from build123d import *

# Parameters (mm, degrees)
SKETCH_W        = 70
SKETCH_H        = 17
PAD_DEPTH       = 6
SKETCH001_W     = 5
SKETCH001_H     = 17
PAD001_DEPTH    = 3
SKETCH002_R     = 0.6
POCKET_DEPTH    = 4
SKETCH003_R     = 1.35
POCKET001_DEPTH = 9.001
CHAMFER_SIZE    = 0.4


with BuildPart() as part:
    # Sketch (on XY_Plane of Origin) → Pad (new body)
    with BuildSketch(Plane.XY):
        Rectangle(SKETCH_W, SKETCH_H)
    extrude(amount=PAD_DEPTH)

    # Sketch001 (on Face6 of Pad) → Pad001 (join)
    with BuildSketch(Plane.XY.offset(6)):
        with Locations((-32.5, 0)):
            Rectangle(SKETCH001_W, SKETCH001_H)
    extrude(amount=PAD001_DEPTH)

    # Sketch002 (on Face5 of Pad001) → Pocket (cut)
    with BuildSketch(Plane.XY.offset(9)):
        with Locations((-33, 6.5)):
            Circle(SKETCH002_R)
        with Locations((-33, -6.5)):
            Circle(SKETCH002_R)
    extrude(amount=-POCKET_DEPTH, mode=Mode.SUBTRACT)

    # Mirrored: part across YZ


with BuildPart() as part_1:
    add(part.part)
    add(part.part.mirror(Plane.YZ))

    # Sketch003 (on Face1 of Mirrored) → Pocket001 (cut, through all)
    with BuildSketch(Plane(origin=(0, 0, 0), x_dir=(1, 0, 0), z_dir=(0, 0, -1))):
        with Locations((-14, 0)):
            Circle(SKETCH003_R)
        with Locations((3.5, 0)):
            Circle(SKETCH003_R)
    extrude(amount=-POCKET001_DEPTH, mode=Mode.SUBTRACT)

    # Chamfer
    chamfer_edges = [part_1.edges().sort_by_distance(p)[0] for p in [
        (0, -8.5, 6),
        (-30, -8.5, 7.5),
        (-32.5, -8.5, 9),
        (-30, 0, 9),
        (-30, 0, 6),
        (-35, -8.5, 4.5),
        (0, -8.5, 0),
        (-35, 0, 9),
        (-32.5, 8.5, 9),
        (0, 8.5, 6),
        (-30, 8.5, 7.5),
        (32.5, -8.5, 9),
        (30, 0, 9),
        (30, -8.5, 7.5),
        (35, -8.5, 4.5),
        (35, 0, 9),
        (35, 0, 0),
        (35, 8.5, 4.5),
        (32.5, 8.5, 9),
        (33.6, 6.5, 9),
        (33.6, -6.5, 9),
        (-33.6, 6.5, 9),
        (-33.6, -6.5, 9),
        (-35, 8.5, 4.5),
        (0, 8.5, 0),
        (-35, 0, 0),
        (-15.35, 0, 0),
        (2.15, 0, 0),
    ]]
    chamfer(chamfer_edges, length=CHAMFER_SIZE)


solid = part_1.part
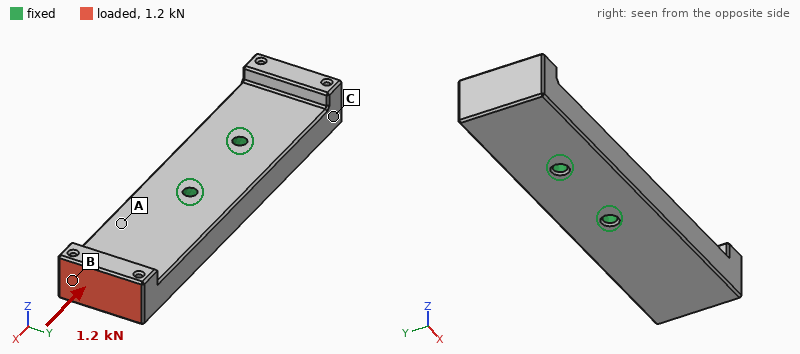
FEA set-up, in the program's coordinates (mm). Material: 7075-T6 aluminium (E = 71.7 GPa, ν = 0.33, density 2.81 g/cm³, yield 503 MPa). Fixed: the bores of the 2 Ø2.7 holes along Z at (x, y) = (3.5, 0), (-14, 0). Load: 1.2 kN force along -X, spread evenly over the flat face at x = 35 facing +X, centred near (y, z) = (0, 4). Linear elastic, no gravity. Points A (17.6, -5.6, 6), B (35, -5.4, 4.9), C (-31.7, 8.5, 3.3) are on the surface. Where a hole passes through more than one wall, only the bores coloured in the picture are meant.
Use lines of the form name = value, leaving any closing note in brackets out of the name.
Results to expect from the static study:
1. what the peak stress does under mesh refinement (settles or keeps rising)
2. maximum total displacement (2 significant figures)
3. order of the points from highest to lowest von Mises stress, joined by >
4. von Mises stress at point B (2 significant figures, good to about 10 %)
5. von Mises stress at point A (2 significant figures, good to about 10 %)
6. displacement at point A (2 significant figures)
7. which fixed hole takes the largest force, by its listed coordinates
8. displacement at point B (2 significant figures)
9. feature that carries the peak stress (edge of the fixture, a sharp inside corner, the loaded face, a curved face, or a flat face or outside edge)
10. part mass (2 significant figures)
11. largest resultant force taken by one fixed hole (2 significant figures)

what the peak stress does under mesh refinement = keeps rising
maximum total displacement = 48 µm
order of the points from highest to lowest von Mises stress, joined by > = A > B > C
von Mises stress at point B = 13 MPa
von Mises stress at point A = 29 MPa
displacement at point A = 12 µm
which fixed hole takes the largest force, by its listed coordinates = (3.5, 0)
displacement at point B = 44 µm
feature that carries the peak stress = edge of the fixture
part mass = 21 g
largest resultant force taken by one fixed hole = 980 N
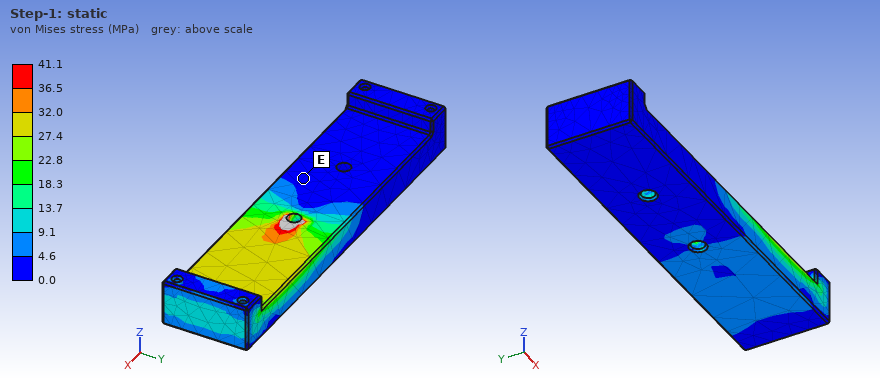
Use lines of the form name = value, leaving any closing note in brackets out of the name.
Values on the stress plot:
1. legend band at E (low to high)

legend band at E = 0.0 to 4.6 MPa
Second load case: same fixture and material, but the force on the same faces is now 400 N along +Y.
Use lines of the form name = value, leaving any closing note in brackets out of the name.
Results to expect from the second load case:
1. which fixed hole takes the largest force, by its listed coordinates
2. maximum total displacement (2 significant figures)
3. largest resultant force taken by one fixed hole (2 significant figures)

which fixed hole takes the largest force, by its listed coordinates = (3.5, 0)
maximum total displacement = 55 µm
largest resultant force taken by one fixed hole = 980 N
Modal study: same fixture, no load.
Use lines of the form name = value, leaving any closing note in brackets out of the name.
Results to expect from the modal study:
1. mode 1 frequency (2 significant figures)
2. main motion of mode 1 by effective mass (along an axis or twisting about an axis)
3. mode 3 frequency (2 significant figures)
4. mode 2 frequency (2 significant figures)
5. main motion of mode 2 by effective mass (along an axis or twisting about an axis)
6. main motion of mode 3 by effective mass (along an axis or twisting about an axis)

mode 1 frequency = 4000 Hz
main motion of mode 1 by effective mass = along Z
mode 3 frequency = 8300 Hz
mode 2 frequency = 7800 Hz
main motion of mode 2 by effective mass = along Y
main motion of mode 3 by effective mass = along Z
